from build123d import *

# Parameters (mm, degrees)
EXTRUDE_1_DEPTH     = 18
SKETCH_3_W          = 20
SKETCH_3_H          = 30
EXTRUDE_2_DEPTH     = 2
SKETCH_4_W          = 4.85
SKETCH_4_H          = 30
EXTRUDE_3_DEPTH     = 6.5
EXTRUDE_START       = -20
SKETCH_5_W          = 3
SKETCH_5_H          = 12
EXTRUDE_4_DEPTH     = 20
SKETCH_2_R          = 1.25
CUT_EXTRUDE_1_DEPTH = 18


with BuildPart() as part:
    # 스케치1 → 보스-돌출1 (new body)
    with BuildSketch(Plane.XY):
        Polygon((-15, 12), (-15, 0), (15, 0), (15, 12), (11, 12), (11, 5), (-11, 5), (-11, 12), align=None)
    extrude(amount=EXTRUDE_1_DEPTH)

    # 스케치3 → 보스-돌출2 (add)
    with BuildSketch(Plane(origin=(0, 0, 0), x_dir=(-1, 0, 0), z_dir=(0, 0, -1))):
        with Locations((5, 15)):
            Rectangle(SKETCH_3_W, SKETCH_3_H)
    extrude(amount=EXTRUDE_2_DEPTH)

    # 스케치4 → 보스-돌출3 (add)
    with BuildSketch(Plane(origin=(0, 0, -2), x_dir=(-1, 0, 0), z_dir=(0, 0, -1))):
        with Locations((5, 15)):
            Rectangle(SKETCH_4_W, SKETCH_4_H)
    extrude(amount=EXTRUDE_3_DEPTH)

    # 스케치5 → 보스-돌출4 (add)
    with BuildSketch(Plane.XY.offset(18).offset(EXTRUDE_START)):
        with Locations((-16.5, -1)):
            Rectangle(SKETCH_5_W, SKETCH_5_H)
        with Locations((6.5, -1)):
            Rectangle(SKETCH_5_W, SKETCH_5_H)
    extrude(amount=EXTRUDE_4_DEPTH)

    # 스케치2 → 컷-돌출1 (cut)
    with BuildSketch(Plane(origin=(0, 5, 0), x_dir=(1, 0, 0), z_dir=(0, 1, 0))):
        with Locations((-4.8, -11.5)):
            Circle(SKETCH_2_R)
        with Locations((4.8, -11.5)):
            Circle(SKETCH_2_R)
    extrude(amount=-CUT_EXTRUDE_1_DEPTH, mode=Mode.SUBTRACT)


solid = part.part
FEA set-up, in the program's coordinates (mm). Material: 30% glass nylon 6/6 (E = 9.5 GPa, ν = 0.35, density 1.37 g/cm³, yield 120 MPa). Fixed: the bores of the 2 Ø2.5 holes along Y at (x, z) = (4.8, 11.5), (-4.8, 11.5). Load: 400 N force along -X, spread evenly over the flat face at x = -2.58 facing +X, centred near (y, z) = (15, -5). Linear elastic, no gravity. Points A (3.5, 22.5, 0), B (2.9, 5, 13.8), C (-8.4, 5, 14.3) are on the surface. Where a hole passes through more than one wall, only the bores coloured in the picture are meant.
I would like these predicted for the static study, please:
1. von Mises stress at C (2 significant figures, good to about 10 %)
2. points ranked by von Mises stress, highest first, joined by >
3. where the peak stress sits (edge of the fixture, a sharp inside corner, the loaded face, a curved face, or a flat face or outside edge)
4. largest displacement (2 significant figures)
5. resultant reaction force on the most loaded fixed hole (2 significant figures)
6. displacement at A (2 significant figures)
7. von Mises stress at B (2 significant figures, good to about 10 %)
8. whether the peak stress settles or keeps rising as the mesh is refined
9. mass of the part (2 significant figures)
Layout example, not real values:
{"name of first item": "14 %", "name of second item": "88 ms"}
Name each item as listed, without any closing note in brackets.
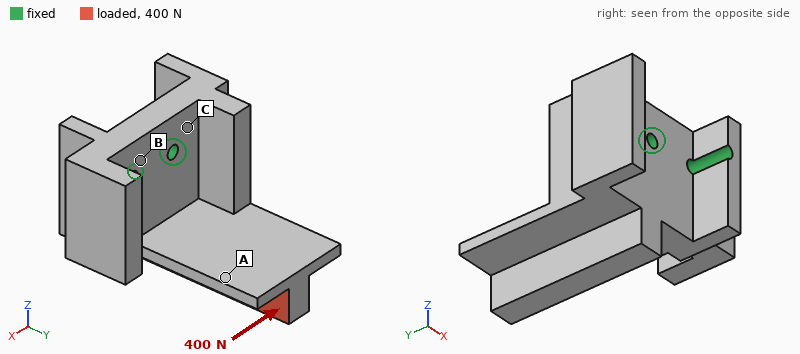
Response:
{"von Mises stress at C": "20 MPa", "points ranked by von Mises stress, highest first, joined by >": "C > B > A", "where the peak stress sits": "edge of the fixture", "largest displacement": "0.55 mm", "resultant reaction force on the most loaded fixed hole": "670 N", "displacement at A": "0.37 mm", "von Mises stress at B": "12 MPa", "whether the peak stress settles or keeps rising as the mesh is refined": "keeps rising", "mass of the part": "9.5 g"}
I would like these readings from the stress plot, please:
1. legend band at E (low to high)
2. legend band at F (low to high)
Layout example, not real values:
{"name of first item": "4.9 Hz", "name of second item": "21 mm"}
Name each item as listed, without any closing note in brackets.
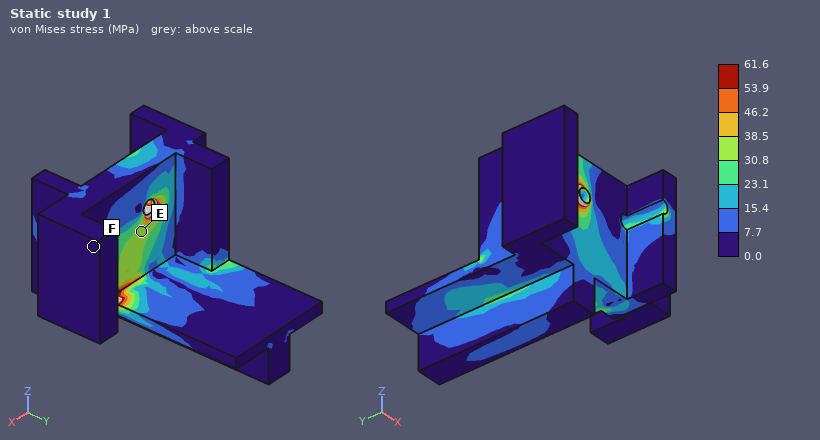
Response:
{"legend band at E": "30.8 to 38.5 MPa", "legend band at F": "0.0 to 7.7 MPa"}
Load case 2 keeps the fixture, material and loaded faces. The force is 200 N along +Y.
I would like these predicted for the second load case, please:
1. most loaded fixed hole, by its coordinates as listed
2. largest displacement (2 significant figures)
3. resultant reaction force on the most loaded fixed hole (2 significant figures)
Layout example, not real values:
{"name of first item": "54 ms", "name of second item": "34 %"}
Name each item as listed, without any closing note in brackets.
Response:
{"most loaded fixed hole, by its coordinates as listed": "(-4.8, 11.5)", "largest displacement": "0.33 mm", "resultant reaction force on the most loaded fixed hole": "120 N"}
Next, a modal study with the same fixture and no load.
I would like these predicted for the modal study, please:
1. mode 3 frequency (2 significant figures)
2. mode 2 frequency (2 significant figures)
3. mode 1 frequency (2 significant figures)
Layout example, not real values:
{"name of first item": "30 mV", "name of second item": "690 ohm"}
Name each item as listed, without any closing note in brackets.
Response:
{"mode 3 frequency": "5800 Hz", "mode 2 frequency": "3400 Hz", "mode 1 frequency": "2000 Hz"}
